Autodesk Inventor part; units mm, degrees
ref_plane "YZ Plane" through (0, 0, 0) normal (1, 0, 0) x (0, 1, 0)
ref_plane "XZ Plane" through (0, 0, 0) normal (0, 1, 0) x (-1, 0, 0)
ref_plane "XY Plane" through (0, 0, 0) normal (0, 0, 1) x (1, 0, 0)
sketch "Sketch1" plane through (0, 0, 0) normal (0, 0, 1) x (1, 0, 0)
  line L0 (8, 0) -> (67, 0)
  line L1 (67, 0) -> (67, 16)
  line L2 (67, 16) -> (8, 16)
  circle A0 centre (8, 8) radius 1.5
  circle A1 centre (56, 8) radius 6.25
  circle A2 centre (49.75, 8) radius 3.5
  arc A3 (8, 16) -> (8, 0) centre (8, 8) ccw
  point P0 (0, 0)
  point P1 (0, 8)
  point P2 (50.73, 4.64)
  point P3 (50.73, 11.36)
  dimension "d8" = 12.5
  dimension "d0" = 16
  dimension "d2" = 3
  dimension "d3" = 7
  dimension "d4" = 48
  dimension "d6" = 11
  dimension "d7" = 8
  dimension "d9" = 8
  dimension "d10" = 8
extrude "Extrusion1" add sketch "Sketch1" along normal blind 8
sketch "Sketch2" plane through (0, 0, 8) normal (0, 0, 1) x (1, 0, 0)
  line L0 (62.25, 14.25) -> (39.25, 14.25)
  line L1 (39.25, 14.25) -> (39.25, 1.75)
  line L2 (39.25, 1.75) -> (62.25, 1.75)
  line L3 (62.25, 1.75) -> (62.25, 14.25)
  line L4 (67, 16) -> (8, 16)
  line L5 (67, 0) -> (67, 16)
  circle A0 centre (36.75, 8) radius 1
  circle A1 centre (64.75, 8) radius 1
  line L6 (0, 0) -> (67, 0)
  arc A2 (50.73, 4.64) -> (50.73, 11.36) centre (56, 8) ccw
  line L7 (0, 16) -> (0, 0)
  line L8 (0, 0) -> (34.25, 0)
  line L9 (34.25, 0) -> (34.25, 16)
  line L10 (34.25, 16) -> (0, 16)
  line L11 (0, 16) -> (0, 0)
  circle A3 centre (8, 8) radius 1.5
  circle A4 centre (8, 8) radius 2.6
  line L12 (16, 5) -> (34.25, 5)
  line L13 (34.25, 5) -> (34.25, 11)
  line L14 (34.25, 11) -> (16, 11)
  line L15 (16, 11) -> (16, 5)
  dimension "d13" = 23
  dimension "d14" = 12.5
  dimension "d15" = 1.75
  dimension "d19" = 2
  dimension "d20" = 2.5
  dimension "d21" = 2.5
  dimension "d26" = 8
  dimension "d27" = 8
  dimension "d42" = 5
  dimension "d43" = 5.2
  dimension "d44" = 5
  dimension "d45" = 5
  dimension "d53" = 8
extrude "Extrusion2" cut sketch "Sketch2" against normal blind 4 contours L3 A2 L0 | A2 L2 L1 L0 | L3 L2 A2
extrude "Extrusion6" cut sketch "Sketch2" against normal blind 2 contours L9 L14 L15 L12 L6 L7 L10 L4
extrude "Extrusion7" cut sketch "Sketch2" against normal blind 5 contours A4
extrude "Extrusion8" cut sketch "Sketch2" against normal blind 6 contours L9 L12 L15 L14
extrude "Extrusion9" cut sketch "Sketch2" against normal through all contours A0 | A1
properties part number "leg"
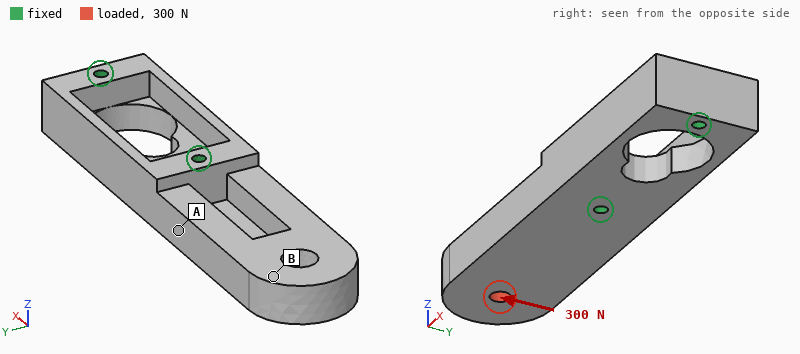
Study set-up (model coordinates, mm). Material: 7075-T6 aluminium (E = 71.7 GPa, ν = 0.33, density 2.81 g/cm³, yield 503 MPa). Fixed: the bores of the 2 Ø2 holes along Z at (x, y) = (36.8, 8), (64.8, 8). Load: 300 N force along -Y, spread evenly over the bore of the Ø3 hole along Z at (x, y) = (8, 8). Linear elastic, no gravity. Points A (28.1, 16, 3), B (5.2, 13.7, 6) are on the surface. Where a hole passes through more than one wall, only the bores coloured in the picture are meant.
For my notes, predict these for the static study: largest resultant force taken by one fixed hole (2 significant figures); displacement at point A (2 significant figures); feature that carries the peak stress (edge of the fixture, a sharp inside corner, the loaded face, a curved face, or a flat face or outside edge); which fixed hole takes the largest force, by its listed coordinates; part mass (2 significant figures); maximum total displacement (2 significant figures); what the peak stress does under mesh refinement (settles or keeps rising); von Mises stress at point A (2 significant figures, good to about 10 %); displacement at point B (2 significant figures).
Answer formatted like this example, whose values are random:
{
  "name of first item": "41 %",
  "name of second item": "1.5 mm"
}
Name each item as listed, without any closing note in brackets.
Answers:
{
  "largest resultant force taken by one fixed hole": "440 N",
  "displacement at point A": "23 µm",
  "feature that carries the peak stress": "edge of the fixture",
  "which fixed hole takes the largest force, by its listed coordinates": "(36.8, 8)",
  "part mass": "14 g",
  "maximum total displacement": "83 µm",
  "what the peak stress does under mesh refinement": "keeps rising",
  "von Mises stress at point A": "26 MPa",
  "displacement at point B": "73 µm"
}
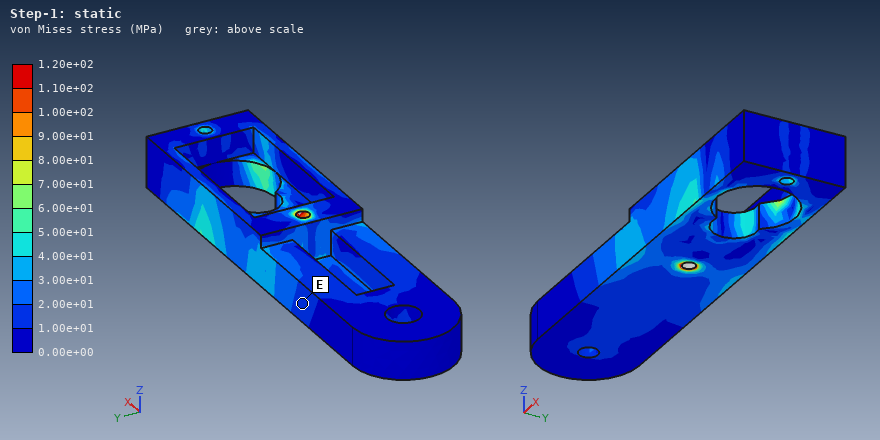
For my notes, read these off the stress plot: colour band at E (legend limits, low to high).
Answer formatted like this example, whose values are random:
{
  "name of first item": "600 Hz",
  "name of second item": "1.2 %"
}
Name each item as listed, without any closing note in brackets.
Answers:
{
  "colour band at E": "1.00e+01 to 2.00e+01 MPa"
}
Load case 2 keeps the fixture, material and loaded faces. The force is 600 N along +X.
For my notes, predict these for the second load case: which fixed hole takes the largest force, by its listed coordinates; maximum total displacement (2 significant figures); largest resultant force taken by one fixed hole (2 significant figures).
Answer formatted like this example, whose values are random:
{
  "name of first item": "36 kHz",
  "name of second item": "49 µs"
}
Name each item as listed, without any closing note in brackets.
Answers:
{
  "which fixed hole takes the largest force, by its listed coordinates": "(36.8, 8)",
  "maximum total displacement": "31 µm",
  "largest resultant force taken by one fixed hole": "560 N"
}
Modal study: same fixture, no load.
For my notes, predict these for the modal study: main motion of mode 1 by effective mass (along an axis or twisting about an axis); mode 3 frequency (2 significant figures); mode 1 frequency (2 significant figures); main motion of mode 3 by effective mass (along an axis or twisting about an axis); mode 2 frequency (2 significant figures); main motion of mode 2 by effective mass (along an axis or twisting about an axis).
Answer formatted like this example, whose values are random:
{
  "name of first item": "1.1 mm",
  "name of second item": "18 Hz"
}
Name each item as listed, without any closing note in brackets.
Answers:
{
  "main motion of mode 1 by effective mass": "along Z",
  "mode 3 frequency": "11 kHz",
  "mode 1 frequency": "3400 Hz",
  "main motion of mode 3 by effective mass": "twisting about X",
  "mode 2 frequency": "5100 Hz",
  "main motion of mode 2 by effective mass": "along Y"
}
